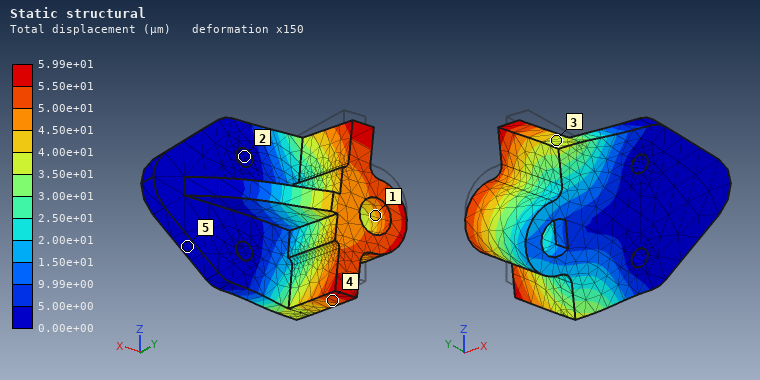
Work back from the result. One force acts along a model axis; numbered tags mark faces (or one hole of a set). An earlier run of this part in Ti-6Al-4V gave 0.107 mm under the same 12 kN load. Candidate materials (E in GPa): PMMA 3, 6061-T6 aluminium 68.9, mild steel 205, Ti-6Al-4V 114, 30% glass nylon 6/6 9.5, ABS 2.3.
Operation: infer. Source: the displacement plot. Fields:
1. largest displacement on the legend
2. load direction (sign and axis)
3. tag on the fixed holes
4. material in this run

5.99e+01 µm
-Z
2
mild steel
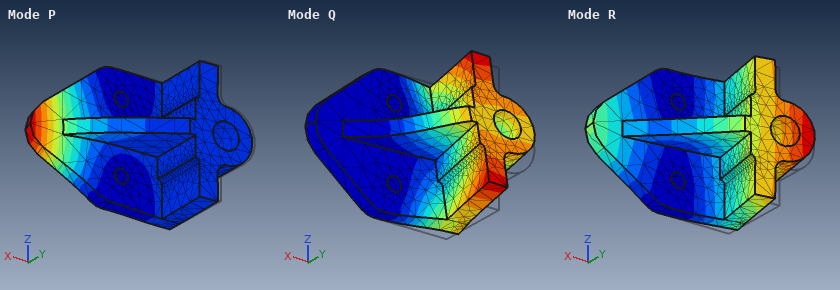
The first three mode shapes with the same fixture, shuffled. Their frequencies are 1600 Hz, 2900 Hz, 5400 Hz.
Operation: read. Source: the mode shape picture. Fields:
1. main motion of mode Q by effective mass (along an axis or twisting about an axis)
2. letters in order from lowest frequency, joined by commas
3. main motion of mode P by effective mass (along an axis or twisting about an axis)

along Z
R, Q, P
along Y
